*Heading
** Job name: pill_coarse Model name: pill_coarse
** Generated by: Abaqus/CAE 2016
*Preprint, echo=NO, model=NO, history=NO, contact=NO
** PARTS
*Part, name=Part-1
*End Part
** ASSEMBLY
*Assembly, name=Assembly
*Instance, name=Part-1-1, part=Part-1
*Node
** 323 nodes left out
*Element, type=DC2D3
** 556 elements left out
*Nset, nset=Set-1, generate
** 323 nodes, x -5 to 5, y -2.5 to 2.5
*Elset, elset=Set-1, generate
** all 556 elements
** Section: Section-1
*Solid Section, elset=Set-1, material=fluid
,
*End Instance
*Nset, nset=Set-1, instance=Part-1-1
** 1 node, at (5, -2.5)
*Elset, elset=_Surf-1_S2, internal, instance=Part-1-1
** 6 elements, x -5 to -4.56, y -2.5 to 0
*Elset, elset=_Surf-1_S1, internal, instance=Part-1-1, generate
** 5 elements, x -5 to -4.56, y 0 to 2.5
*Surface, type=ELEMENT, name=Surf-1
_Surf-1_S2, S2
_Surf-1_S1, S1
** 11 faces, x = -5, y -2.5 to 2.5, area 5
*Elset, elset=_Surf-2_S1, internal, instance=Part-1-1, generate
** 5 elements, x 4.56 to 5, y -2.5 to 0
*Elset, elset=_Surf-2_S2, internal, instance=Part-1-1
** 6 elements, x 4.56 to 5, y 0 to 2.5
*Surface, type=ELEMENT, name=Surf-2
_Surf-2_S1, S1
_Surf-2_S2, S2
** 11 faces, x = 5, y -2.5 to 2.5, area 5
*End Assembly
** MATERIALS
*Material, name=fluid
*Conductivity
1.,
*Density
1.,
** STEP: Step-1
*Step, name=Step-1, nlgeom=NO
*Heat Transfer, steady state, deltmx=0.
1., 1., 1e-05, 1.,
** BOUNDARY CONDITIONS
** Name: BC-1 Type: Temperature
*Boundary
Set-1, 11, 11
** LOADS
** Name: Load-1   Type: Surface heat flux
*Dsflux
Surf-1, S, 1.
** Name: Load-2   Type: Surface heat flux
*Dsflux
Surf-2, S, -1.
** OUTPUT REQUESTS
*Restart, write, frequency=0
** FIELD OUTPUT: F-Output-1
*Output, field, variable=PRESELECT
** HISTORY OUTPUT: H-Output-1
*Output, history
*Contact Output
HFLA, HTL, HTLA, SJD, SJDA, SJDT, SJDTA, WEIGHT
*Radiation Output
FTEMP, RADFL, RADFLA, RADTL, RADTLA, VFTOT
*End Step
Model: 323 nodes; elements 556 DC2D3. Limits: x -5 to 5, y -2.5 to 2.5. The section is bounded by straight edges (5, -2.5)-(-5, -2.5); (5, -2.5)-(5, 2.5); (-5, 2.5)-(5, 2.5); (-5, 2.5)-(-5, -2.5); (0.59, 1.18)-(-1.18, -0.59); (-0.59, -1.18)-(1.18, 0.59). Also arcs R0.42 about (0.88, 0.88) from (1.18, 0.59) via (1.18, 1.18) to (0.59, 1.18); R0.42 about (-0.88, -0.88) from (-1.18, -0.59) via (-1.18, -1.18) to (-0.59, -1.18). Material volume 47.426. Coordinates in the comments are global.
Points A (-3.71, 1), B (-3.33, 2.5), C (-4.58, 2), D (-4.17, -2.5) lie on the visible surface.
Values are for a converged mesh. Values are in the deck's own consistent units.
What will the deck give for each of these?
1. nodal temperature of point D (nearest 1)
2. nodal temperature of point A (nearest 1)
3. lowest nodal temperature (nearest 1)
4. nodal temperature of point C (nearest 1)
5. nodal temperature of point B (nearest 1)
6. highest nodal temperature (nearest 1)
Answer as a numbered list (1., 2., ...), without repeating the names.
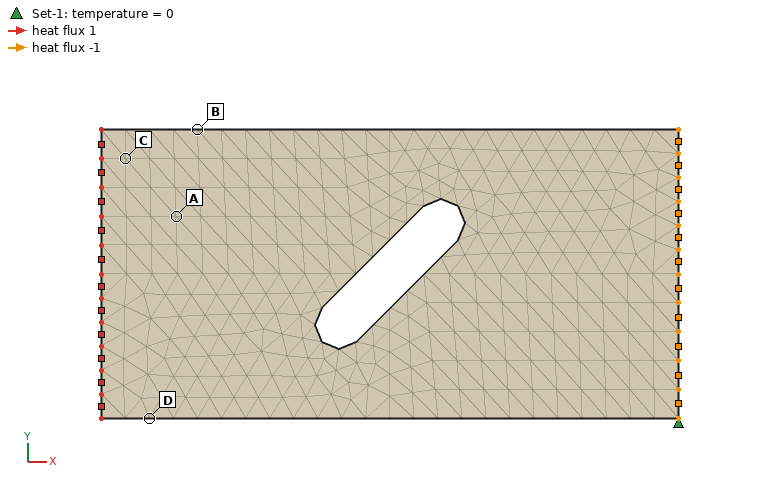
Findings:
1. 11
2. 11
3. 0
4. 12
5. 10
6. 12
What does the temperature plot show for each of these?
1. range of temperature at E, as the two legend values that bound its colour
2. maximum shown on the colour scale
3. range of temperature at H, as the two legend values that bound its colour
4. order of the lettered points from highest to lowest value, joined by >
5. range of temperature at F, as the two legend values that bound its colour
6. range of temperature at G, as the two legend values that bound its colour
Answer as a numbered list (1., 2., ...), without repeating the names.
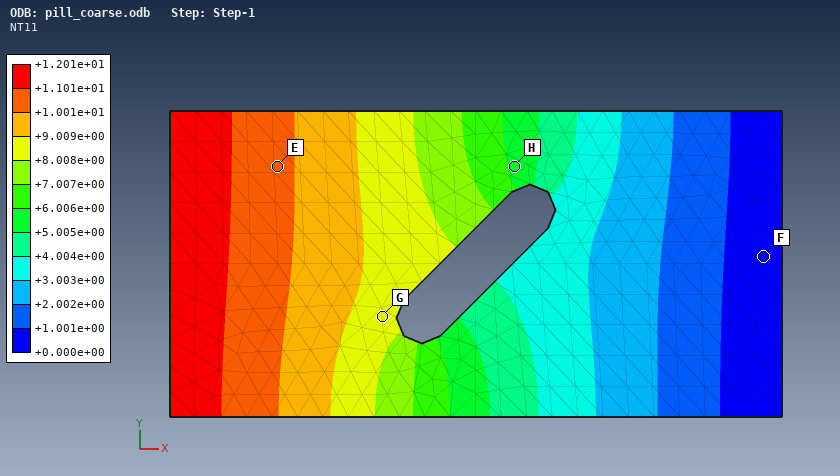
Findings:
1. +1.001e+01 to +1.101e+01
2. +1.201e+01
3. +5.005e+00 to +6.006e+00
4. E > G > H > F
5. +0.000e+00 to +1.001e+00
6. +8.008e+00 to +9.009e+00
